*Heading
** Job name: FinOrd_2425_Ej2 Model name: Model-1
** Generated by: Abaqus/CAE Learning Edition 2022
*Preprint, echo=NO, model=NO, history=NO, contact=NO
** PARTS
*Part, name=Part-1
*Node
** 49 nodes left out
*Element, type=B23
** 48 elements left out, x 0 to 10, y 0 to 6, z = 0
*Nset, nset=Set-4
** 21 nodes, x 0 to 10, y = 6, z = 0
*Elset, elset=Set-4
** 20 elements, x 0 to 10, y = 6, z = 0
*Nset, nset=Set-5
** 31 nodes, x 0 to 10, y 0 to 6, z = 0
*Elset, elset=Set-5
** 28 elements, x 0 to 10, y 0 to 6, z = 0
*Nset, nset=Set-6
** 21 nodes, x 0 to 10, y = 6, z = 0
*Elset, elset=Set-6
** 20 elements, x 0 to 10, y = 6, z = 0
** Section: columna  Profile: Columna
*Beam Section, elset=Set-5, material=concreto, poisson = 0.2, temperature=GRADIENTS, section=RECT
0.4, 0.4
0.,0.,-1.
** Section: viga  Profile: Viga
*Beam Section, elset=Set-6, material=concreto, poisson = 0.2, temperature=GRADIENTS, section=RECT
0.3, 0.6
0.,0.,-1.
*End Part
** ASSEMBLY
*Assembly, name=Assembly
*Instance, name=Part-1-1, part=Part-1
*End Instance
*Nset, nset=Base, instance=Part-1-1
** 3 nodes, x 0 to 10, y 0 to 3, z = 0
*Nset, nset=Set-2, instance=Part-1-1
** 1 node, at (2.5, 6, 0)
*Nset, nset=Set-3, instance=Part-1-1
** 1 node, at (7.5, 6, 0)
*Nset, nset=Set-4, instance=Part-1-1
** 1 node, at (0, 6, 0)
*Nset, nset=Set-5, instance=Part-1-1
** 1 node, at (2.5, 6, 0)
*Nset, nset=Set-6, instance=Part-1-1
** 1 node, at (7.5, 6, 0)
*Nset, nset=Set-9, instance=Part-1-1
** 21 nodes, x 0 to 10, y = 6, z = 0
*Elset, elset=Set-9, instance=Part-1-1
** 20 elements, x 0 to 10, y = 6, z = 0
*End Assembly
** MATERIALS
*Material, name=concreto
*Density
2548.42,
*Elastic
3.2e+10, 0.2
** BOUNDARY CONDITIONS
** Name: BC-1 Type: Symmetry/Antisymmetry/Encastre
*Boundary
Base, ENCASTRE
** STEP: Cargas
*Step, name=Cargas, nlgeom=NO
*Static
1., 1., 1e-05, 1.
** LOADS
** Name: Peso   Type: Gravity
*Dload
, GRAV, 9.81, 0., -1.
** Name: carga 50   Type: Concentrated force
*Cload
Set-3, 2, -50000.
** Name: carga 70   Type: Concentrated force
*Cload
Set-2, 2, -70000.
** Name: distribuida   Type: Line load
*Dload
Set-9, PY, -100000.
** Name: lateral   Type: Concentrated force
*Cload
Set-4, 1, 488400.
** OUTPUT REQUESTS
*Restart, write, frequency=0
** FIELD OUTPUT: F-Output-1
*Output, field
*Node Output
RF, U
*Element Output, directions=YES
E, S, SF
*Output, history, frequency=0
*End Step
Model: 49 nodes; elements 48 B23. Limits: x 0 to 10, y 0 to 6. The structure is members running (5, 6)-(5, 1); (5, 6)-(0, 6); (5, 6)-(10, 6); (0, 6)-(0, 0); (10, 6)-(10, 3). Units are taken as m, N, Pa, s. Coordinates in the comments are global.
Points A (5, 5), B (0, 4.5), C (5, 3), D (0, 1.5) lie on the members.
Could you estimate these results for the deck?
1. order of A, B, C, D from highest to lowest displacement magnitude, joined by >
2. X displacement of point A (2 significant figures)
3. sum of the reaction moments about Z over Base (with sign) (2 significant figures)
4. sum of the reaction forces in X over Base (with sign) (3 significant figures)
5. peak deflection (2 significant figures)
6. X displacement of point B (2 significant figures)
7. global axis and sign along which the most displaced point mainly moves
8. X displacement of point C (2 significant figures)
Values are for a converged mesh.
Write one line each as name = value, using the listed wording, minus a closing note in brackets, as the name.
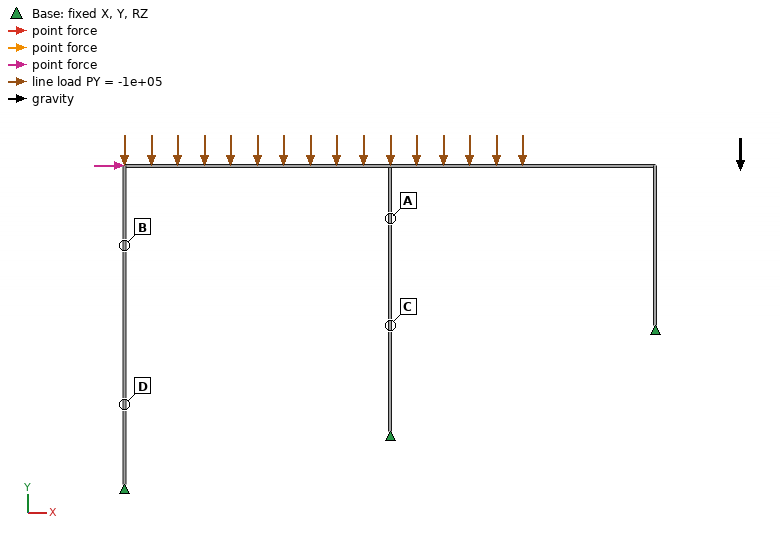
order of A, B, C, D from highest to lowest displacement magnitude, joined by > = A > B > C > D
X displacement of point A = 0.013 m
sum of the reaction moments about Z over Base (with sign) = 9.4e+05 N·m
sum of the reaction forces in X over Base (with sign) = -4.88e+05 N
peak deflection = 0.015 m
X displacement of point B = 0.011 m
global axis and sign along which the most displaced point mainly moves = +X
X displacement of point C = 0.0053 m
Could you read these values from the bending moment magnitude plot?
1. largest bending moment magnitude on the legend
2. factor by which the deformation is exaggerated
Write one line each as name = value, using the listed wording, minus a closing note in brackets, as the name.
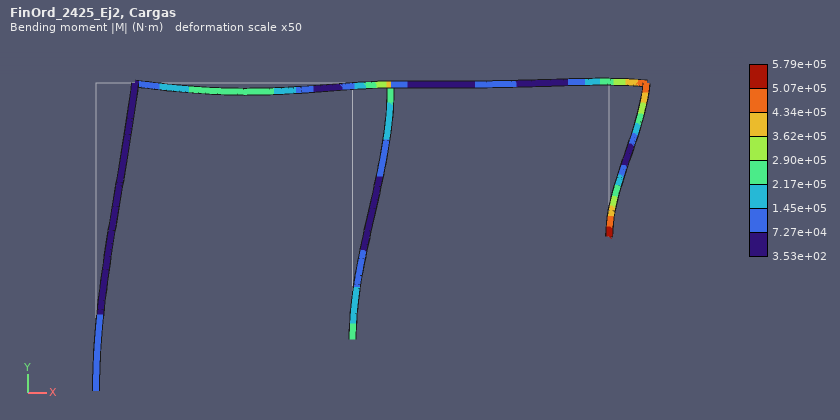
largest bending moment magnitude on the legend = 5.79e+05 N·m
factor by which the deformation is exaggerated = 50
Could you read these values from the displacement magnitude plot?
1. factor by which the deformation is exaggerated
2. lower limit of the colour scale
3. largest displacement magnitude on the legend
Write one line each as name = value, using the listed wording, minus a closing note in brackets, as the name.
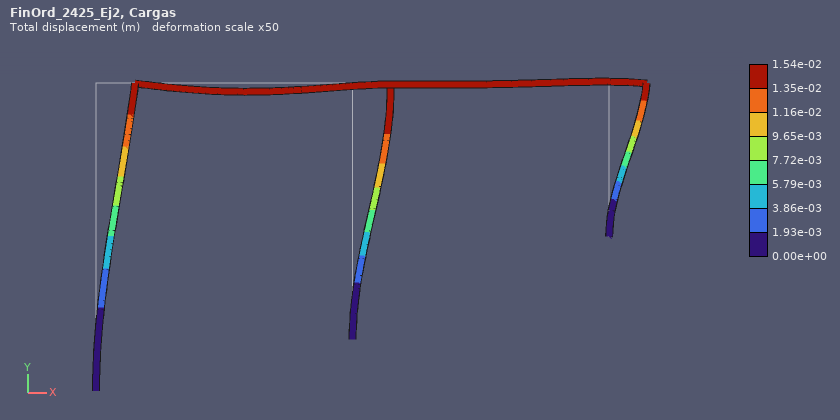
factor by which the deformation is exaggerated = 50
lower limit of the colour scale = 0.00e+00 m
largest displacement magnitude on the legend = 1.54e-02 m
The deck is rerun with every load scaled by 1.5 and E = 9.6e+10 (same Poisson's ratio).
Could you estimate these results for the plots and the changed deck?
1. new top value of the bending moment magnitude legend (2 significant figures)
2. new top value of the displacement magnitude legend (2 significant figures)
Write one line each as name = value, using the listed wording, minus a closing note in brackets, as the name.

new top value of the bending moment magnitude legend = 8.7e+05 N·m
new top value of the displacement magnitude legend = 0.0077 m
